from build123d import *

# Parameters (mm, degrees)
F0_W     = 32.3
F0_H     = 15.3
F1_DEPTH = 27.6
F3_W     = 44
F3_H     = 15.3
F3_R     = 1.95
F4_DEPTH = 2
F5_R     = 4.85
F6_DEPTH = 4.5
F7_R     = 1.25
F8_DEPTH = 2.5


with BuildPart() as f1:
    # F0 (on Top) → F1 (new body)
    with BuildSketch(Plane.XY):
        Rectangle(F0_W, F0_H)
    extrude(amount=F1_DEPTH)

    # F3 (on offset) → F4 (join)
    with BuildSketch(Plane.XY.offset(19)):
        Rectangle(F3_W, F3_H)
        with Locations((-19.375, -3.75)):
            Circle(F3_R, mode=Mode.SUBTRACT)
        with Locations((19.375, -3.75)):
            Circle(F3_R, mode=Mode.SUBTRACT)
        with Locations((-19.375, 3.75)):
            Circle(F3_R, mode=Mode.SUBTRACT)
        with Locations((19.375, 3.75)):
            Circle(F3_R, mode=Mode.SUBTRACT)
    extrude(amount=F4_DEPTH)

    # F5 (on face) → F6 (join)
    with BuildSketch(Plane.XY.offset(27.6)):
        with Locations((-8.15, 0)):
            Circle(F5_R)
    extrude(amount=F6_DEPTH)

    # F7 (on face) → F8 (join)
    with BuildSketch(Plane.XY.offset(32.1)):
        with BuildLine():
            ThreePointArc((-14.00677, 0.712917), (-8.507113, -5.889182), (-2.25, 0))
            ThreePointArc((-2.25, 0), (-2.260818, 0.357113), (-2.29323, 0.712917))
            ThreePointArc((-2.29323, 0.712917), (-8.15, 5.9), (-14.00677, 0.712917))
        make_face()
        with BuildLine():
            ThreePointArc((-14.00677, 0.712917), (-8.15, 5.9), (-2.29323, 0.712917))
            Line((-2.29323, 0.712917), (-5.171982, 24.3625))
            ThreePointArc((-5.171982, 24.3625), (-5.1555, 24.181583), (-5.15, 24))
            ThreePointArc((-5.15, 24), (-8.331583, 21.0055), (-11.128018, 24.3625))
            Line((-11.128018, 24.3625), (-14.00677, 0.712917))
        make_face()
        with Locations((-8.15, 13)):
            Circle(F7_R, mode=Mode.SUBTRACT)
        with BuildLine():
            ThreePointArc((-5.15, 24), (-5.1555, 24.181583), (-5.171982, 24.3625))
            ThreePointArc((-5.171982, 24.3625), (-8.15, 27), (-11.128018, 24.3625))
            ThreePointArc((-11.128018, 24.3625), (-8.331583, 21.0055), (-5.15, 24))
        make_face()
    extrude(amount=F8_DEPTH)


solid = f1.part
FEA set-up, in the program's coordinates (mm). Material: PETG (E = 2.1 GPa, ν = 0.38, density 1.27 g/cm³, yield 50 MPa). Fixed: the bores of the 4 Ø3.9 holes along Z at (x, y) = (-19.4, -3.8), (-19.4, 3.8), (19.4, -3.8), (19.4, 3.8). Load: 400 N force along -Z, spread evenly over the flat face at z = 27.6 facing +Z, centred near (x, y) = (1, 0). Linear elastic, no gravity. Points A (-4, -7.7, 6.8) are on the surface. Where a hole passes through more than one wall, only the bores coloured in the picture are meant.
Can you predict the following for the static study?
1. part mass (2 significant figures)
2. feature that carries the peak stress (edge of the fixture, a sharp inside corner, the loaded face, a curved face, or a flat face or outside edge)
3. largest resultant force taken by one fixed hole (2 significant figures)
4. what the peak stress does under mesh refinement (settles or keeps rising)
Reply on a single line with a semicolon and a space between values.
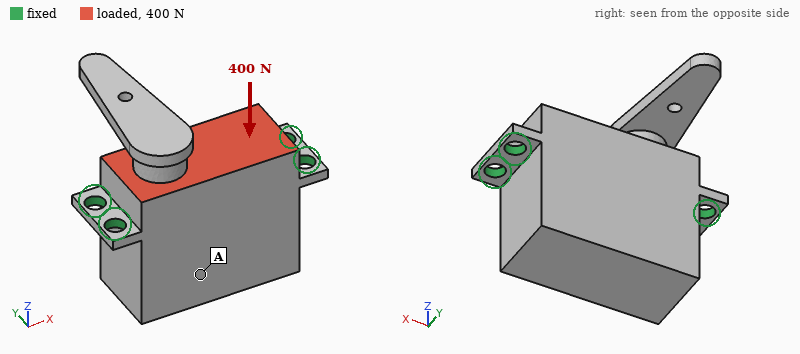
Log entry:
19 g; edge of the fixture; 110 N; keeps rising
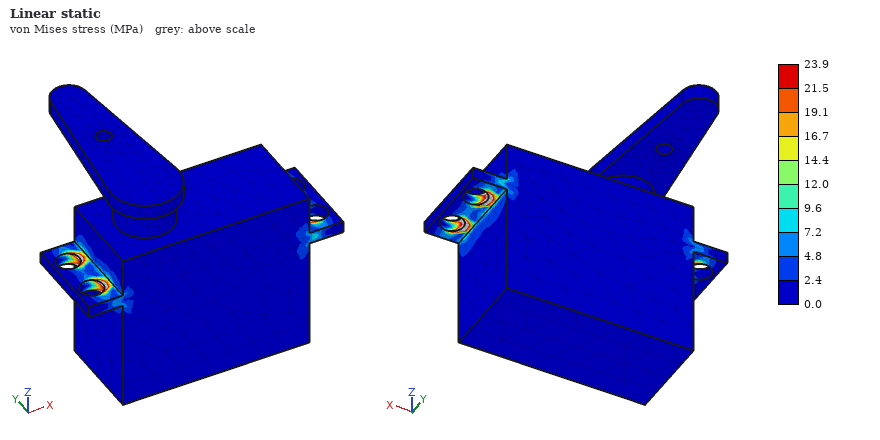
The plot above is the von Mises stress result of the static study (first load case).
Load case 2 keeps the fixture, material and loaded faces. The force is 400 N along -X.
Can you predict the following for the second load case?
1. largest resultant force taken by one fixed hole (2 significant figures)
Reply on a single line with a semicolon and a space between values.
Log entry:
110 N
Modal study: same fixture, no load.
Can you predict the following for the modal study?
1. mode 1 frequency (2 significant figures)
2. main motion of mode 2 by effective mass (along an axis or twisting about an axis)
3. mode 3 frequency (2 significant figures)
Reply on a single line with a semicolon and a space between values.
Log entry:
1100 Hz; along Y; 2700 Hz
